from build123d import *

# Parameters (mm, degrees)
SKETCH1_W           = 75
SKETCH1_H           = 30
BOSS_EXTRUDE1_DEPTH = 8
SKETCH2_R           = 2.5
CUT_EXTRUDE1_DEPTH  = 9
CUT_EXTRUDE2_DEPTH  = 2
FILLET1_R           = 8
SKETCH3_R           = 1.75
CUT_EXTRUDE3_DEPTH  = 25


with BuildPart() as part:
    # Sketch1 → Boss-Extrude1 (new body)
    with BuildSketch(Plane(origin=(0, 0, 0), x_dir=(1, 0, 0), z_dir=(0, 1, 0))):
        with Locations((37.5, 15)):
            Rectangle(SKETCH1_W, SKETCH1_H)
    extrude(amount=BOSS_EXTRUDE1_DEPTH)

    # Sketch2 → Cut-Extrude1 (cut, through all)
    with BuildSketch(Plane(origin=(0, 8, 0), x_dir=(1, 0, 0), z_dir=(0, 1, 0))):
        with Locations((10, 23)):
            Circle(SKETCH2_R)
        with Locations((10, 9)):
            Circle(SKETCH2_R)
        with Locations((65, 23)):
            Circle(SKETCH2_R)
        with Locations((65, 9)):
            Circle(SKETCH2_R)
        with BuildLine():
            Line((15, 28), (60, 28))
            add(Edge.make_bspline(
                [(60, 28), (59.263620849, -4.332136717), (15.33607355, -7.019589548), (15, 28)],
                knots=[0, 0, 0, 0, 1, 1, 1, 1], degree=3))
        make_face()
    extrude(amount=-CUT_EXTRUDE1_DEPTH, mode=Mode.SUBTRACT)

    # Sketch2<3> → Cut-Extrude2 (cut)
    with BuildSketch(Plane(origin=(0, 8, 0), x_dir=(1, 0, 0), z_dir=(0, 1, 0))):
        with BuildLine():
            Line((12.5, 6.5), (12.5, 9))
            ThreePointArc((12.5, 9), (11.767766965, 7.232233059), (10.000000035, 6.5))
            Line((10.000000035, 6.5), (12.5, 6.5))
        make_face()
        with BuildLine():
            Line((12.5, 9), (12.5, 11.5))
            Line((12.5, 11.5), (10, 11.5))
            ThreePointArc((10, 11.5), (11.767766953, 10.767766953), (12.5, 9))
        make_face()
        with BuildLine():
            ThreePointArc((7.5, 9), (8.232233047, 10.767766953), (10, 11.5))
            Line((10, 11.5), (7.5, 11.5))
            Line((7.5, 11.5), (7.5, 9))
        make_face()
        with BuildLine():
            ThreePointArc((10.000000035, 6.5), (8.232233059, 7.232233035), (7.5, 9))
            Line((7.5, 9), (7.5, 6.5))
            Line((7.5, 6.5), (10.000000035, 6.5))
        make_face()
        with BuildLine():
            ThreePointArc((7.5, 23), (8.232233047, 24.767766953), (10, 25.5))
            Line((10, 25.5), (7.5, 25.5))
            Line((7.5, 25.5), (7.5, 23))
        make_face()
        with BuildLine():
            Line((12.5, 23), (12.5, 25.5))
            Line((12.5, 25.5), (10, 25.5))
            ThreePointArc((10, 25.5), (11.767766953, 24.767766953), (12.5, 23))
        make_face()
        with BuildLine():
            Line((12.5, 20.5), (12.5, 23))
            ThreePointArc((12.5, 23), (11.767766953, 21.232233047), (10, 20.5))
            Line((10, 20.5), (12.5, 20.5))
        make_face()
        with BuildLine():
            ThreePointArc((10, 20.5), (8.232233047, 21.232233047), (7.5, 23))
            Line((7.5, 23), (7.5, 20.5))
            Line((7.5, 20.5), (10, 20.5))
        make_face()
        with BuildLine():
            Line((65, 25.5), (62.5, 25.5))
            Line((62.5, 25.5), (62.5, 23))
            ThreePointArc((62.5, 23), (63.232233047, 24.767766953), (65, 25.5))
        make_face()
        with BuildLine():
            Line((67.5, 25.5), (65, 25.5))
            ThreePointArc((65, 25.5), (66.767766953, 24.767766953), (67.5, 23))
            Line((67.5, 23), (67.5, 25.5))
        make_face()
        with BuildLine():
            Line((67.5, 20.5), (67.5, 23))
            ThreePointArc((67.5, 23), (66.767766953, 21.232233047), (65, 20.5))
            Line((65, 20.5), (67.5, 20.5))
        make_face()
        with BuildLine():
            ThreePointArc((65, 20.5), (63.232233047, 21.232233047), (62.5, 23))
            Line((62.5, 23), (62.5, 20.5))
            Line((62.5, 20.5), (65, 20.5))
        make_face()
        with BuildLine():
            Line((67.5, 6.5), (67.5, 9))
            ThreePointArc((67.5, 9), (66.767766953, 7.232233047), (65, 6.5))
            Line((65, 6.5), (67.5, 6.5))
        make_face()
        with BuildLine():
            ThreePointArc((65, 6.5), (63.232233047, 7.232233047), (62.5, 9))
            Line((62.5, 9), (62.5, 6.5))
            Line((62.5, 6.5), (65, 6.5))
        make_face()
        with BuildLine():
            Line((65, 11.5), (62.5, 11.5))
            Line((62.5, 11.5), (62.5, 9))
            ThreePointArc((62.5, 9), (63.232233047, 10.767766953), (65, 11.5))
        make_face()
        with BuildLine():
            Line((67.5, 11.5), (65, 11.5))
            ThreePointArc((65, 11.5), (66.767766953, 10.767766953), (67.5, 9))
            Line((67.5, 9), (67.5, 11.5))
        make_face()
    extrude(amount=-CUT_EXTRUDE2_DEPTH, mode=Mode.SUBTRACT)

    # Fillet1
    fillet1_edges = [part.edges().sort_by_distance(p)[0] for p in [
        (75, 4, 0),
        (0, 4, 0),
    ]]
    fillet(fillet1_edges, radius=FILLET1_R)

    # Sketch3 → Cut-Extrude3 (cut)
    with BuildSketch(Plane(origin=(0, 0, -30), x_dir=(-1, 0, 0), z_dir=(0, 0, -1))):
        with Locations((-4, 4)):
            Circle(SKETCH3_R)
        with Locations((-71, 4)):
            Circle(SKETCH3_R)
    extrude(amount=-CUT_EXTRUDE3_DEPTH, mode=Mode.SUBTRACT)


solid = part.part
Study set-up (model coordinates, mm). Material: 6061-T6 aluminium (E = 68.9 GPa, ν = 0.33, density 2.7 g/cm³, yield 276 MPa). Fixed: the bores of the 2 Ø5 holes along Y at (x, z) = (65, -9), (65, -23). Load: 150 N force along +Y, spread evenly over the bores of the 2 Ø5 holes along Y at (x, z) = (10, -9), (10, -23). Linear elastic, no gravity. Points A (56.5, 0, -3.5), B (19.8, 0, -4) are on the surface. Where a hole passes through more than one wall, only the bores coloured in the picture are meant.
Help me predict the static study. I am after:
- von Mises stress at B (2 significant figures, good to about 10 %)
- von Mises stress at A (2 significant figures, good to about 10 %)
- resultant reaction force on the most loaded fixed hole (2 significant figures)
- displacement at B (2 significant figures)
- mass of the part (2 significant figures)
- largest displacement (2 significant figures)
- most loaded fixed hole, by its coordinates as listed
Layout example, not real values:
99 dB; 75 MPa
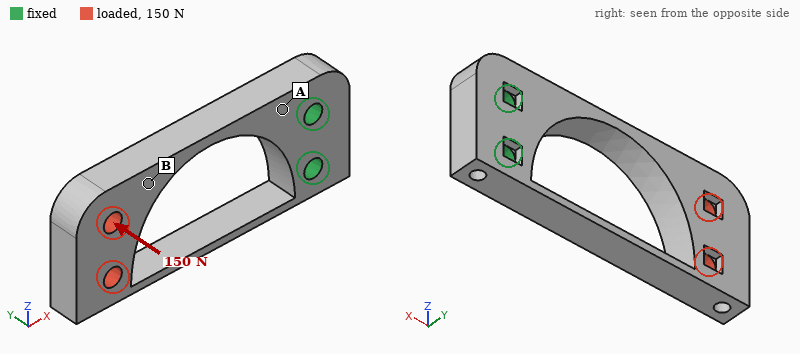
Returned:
16 MPa; 41 MPa; 100 N; 0.24 mm; 25 g; 0.55 mm; (65, -9)
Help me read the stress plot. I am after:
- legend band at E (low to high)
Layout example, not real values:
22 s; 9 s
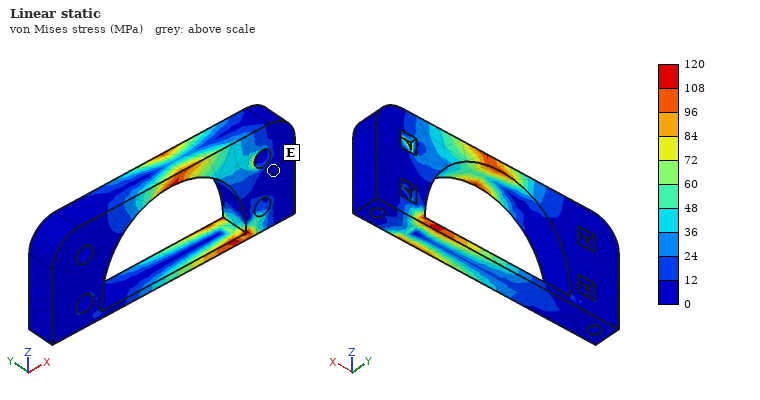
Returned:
0 to 12 MPa
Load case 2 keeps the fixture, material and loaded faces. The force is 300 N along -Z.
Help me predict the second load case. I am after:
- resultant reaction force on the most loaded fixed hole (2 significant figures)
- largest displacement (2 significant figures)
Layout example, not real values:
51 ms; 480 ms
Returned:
860 N; 0.21 mm
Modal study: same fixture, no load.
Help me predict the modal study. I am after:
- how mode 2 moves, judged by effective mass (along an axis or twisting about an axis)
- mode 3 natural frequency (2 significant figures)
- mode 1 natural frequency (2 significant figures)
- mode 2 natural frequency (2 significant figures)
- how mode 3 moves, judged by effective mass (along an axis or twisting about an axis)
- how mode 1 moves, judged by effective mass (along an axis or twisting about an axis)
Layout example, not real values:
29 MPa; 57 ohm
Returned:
along Z; 3000 Hz; 950 Hz; 1800 Hz; twisting about X; along Y
